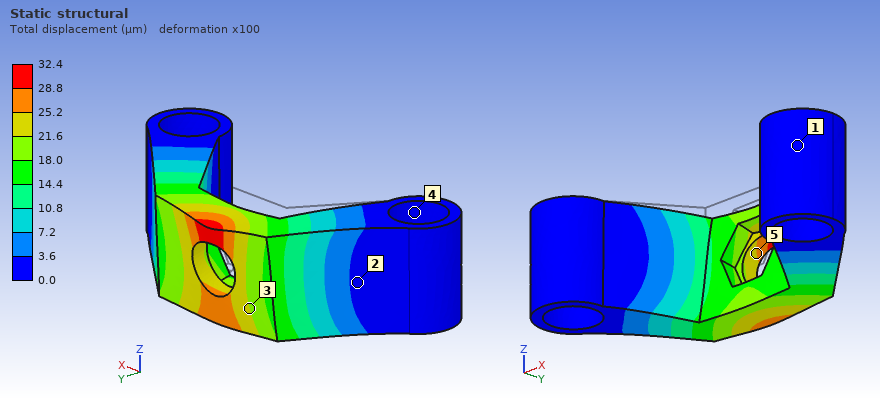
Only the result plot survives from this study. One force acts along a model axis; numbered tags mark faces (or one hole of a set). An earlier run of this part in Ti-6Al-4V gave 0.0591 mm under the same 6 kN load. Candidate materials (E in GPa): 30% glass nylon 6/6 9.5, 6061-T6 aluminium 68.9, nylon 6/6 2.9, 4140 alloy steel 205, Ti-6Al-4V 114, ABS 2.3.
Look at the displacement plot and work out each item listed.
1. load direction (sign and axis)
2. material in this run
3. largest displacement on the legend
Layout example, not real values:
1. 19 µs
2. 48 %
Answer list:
1. -Z
2. 4140 alloy steel
3. 32.4 µm
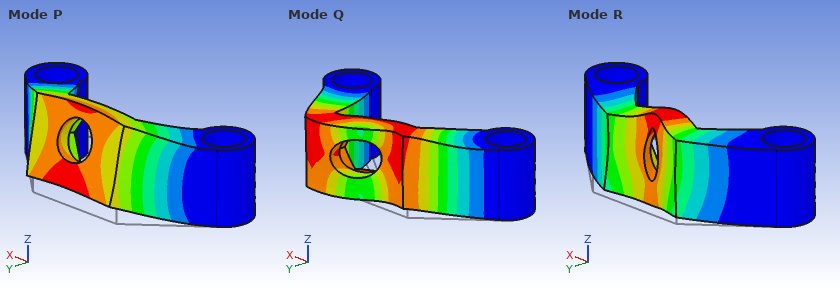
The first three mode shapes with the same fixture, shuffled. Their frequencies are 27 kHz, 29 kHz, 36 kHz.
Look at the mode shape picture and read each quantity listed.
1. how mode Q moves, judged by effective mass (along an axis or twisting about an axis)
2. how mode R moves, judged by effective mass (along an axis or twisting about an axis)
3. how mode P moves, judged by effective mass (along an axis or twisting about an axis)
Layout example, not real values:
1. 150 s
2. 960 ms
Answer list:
1. along X
2. along Y
3. along Z
